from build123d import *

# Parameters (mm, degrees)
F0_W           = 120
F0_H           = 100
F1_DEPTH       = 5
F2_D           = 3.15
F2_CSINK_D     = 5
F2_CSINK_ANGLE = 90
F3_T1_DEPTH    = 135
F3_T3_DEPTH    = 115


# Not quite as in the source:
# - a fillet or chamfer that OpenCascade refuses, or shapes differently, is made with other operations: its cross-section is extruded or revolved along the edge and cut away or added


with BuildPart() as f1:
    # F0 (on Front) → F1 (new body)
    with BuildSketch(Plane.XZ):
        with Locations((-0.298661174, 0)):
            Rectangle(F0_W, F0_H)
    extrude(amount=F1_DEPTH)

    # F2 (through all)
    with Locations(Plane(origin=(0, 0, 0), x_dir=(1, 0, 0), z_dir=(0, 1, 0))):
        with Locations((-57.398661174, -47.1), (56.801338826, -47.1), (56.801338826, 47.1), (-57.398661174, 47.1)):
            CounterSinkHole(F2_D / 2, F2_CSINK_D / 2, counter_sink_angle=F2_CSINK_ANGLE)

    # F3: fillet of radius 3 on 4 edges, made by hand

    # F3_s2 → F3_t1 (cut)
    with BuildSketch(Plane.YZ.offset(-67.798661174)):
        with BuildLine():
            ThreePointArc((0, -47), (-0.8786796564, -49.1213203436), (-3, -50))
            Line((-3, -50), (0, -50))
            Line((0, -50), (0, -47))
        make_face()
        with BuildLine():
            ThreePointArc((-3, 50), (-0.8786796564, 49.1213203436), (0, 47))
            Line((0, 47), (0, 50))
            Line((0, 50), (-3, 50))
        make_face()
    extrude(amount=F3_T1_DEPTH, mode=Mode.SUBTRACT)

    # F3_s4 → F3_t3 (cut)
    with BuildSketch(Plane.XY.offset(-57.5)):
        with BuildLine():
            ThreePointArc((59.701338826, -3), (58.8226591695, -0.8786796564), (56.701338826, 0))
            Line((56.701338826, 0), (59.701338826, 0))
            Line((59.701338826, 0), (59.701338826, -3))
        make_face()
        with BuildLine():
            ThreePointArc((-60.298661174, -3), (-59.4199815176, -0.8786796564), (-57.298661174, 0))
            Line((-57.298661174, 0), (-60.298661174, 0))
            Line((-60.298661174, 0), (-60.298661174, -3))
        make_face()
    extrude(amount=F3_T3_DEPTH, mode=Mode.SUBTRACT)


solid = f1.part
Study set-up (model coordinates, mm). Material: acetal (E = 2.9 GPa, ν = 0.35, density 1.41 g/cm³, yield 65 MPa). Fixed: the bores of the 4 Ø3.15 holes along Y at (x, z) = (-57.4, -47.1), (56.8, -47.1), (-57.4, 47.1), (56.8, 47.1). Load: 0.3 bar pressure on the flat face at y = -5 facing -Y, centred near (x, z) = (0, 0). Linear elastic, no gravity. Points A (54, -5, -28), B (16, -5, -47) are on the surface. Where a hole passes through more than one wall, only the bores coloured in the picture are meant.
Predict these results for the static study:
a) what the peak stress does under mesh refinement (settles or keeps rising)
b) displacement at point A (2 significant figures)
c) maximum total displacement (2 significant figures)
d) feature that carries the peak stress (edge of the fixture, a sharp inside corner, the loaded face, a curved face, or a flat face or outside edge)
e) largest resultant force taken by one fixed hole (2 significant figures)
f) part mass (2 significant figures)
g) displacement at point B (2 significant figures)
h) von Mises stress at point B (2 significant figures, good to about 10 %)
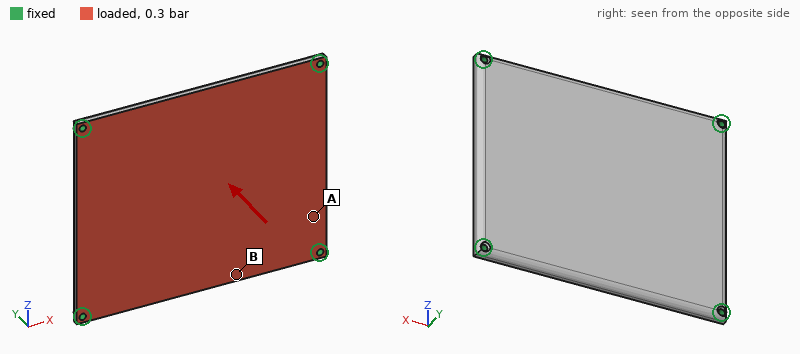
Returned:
keeps rising
0.31 mm
1.3 mm
edge of the fixture
97 N
83 g
0.90 mm
6.3 MPa
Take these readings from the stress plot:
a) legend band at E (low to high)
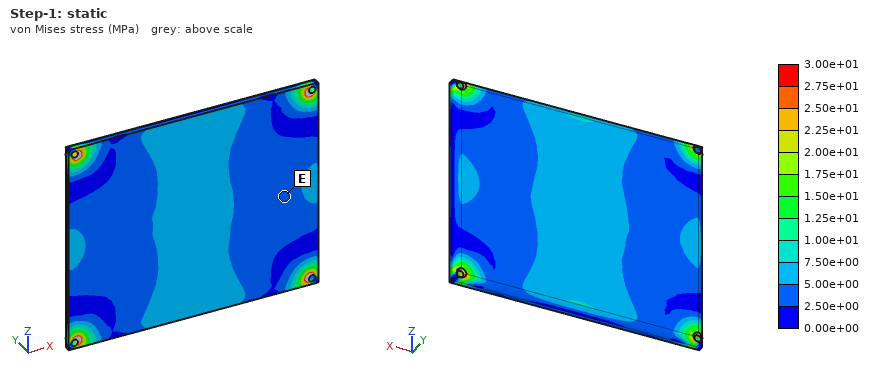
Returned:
2.50e+00 to 5.00e+00 MPa
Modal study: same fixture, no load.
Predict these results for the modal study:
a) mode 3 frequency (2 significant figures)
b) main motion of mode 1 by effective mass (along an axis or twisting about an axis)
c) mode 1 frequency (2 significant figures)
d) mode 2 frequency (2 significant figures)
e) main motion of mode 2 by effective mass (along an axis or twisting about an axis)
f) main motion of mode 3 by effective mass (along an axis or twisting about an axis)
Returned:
720 Hz
along Y
340 Hz
610 Hz
twisting about X
twisting about Z
